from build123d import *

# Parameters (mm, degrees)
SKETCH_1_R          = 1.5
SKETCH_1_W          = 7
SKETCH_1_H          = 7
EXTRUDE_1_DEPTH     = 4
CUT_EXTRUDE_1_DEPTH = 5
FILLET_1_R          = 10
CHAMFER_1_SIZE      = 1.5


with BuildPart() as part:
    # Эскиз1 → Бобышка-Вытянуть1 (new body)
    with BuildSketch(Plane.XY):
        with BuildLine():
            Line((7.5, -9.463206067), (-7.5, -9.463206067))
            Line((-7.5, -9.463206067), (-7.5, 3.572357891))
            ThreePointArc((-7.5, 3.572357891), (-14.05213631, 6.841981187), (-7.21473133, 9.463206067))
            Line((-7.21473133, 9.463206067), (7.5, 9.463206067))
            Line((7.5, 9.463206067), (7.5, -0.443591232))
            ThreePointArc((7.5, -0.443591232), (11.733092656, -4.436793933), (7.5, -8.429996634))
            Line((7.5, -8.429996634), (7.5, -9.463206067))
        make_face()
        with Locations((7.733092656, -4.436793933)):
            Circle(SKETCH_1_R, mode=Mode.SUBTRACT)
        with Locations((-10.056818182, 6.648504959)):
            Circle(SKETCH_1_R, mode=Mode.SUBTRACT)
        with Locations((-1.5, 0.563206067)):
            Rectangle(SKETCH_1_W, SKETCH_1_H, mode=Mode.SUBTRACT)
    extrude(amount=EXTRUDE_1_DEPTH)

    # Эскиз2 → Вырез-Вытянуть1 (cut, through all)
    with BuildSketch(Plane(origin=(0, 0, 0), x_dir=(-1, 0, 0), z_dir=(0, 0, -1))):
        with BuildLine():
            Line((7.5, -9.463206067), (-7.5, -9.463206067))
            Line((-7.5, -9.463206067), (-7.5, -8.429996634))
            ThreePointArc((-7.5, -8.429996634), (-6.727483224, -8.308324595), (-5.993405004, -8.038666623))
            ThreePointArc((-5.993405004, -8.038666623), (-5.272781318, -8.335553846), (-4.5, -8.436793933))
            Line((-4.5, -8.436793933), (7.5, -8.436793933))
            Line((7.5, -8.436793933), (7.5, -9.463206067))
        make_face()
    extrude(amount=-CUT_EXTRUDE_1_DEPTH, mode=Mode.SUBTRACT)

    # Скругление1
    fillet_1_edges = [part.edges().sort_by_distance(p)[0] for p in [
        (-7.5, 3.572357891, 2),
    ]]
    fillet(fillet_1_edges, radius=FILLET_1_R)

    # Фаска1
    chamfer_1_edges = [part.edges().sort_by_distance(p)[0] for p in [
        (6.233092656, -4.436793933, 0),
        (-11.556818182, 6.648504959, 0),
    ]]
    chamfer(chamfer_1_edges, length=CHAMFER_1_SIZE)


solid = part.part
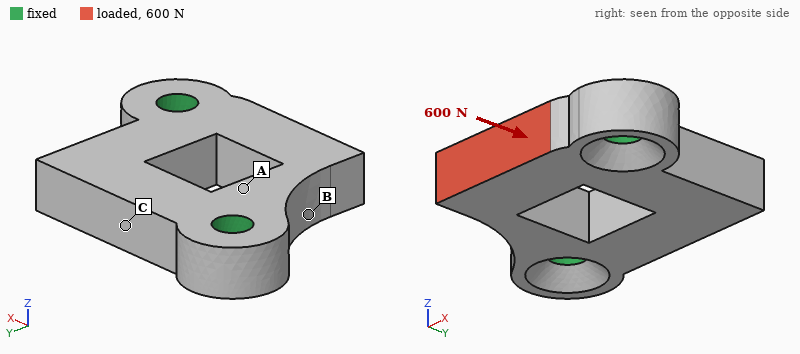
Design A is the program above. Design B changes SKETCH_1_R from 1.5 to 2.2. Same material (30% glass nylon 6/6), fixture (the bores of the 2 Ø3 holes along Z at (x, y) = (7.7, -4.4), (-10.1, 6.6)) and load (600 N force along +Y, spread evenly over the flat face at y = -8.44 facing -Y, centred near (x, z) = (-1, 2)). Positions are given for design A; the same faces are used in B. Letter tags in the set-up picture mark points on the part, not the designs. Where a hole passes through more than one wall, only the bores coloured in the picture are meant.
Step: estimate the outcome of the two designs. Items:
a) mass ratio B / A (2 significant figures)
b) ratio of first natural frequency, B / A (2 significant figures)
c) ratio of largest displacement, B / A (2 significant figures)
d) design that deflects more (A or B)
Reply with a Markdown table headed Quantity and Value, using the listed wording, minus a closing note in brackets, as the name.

| Quantity | Value |
|---|---|
| mass ratio B / A | 0.93 |
| ratio of first natural frequency, B / A | 1.1 |
| ratio of largest displacement, B / A | 0.89 |
| design that deflects more | A |
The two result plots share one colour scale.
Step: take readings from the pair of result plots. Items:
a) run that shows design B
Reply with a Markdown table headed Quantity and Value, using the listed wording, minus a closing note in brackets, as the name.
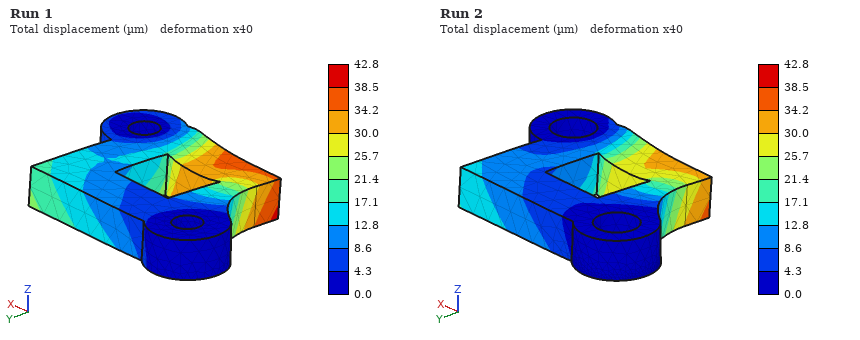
| Quantity | Value |
|---|---|
| run that shows design B | Run 2 |
